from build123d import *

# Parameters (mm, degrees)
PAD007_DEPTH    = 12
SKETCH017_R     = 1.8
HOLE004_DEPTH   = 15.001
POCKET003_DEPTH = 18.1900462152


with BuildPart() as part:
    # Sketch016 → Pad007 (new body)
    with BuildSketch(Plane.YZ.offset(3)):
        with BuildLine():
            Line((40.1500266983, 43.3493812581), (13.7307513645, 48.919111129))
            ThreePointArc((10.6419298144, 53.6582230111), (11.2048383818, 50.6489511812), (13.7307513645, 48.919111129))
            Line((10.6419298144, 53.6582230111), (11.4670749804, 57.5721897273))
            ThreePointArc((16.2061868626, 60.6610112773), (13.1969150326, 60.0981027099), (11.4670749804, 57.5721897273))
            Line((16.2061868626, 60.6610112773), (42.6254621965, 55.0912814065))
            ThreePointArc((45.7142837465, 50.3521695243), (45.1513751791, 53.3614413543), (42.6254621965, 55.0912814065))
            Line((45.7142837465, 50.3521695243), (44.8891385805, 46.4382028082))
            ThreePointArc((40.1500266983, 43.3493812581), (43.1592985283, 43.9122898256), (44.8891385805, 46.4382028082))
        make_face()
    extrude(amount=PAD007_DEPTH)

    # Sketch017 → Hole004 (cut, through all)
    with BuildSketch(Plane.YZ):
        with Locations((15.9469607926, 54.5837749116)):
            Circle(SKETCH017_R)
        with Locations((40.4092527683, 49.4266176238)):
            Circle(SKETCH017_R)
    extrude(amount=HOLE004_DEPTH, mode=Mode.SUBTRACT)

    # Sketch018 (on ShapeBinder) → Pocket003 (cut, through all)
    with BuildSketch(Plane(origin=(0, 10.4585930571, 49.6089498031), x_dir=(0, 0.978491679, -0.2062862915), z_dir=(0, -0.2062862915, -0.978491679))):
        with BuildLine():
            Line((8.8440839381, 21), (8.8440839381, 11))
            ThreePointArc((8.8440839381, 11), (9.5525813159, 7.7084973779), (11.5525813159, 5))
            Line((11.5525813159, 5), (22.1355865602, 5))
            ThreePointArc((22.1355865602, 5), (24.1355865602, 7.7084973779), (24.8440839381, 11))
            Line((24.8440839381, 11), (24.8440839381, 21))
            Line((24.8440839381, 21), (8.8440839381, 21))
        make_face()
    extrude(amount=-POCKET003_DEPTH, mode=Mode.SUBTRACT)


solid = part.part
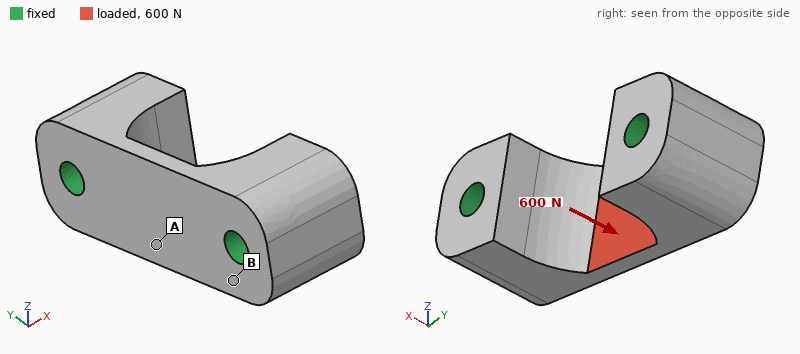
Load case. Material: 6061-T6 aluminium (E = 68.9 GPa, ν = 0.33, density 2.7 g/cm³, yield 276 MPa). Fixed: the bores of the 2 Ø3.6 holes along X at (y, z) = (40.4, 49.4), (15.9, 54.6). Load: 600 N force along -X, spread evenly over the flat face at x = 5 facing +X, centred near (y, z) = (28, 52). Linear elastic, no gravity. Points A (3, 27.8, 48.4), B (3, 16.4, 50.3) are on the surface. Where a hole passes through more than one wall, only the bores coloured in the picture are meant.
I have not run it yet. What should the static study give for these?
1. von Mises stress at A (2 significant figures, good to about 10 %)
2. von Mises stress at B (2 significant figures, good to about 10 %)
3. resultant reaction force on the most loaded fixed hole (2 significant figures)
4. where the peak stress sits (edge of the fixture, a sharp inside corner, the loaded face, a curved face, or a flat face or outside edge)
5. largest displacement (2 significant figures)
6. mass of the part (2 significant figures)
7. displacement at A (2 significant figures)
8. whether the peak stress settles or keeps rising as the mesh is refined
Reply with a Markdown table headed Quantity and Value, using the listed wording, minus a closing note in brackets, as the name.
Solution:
| Quantity | Value |
|---|---|
| von Mises stress at A | 56 MPa |
| von Mises stress at B | 8.3 MPa |
| resultant reaction force on the most loaded fixed hole | 350 N |
| where the peak stress sits | a sharp inside corner |
| largest displacement | 13 µm |
| mass of the part | 7.6 g |
| displacement at A | 12 µm |
| whether the peak stress settles or keeps rising as the mesh is refined | keeps rising |
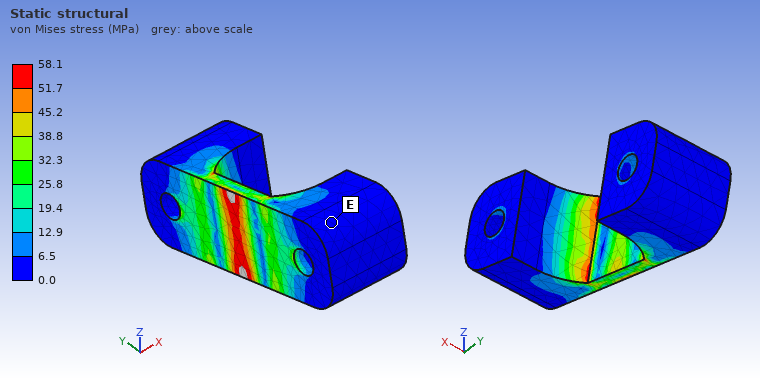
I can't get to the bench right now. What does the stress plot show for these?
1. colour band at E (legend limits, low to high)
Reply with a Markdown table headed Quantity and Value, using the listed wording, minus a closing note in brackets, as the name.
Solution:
| Quantity | Value |
|---|---|
| colour band at E | 0.0 to 6.5 MPa |
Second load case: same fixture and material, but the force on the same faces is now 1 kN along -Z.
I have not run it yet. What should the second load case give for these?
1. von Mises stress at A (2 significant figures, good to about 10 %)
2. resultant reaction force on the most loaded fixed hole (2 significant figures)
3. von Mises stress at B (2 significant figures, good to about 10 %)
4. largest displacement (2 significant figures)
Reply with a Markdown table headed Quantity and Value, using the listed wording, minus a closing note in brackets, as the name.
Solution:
| Quantity | Value |
|---|---|
| von Mises stress at A | 34 MPa |
| resultant reaction force on the most loaded fixed hole | 500 N |
| von Mises stress at B | 8.0 MPa |
| largest displacement | 12 µm |
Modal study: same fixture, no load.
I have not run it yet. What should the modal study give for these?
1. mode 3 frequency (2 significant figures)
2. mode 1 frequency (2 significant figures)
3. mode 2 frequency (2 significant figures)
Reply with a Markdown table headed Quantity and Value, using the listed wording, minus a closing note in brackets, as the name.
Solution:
| Quantity | Value |
|---|---|
| mode 3 frequency | 59 kHz |
| mode 1 frequency | 47 kHz |
| mode 2 frequency | 53 kHz |
